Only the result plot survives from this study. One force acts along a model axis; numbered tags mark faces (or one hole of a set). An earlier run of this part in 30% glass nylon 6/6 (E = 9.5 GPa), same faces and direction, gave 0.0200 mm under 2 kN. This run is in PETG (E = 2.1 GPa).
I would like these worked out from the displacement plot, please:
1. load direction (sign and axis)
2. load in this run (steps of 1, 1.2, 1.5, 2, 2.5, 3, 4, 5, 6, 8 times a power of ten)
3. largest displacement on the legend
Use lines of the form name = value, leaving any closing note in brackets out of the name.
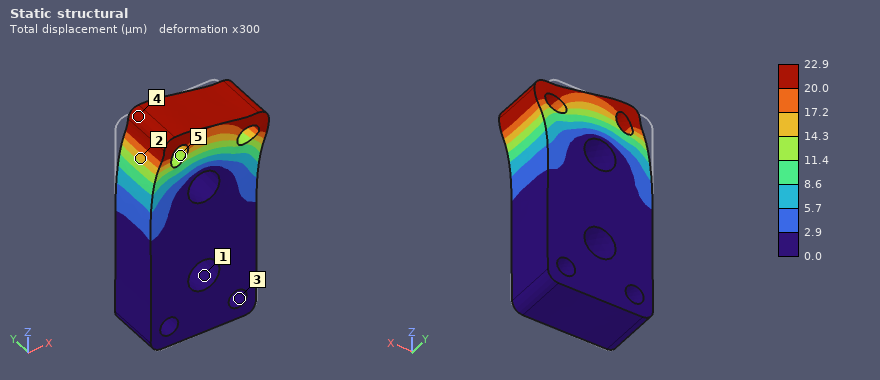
load direction = +X
load in this run = 500 N
largest displacement on the legend = 22.9 µm
